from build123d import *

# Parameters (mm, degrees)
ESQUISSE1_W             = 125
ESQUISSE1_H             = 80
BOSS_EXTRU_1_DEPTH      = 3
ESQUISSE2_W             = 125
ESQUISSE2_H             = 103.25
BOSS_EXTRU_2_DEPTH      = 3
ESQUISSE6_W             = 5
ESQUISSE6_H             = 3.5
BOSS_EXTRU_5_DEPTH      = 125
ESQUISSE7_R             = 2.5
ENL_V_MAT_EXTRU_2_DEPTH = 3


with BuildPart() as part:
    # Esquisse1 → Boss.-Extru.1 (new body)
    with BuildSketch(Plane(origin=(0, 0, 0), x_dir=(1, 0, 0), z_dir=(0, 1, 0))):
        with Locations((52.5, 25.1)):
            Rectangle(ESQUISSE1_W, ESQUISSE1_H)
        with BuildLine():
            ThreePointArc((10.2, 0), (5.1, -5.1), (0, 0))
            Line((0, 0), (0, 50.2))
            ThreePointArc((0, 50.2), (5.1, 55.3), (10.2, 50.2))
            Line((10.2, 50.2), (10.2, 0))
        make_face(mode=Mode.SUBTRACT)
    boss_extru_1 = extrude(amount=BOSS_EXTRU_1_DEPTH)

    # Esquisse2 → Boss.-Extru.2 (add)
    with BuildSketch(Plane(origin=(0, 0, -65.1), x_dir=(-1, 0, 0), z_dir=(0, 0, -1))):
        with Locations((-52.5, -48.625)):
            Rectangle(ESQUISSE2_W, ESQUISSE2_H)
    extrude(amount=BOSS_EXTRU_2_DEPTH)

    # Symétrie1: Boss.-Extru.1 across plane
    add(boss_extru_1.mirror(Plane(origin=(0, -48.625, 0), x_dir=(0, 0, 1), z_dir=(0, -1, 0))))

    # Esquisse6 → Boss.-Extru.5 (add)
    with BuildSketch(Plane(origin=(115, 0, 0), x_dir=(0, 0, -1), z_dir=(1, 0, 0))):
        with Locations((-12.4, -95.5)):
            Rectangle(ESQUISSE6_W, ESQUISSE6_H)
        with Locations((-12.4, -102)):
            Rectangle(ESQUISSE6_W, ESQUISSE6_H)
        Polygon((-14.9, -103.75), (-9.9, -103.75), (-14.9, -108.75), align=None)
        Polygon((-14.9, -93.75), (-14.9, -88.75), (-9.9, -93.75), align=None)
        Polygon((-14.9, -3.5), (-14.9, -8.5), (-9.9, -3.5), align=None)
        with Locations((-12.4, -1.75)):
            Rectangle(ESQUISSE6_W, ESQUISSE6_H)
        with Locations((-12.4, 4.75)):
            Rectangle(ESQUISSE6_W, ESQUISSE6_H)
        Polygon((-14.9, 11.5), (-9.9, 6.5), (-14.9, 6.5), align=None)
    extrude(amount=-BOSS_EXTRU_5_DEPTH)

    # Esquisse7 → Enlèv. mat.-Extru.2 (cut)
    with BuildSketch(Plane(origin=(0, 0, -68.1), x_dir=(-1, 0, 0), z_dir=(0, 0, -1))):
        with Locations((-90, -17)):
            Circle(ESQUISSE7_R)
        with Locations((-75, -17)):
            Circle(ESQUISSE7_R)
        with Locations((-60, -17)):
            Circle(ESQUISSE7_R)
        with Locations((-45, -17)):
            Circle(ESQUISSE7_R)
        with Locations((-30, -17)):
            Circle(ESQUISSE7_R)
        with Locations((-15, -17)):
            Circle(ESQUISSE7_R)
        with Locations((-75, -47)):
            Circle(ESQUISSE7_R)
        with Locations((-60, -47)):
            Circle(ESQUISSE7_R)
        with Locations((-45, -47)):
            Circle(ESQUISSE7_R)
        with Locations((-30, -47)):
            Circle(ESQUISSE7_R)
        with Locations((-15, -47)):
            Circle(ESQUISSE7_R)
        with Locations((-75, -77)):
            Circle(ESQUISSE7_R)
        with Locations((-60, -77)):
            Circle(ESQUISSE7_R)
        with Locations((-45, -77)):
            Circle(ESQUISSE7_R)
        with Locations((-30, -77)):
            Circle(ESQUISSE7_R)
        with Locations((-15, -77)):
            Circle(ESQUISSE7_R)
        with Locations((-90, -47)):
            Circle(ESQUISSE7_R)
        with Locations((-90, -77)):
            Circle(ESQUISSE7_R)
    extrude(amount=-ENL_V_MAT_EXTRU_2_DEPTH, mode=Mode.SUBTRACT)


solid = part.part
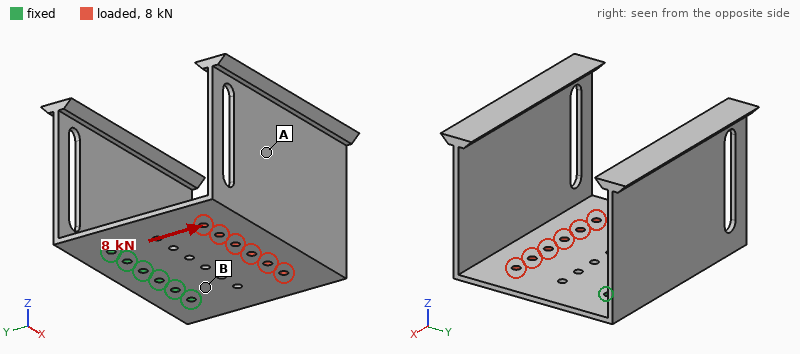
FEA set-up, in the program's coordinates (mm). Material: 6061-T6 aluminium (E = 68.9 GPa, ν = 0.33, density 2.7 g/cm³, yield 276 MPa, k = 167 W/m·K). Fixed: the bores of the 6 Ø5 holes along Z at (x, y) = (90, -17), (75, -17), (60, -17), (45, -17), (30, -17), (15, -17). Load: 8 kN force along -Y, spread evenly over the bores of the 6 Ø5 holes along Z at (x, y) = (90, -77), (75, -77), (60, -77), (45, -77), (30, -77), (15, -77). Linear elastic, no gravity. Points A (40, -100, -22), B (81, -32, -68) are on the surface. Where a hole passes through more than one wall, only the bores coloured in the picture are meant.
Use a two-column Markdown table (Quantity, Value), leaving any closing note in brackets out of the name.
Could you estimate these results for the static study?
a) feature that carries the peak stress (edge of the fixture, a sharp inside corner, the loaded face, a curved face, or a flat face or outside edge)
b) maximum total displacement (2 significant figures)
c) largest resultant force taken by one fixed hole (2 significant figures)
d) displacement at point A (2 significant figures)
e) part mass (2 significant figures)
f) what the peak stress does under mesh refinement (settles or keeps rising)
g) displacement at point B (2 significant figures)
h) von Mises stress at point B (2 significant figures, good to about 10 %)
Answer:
| Quantity | Value |
|---|---|
| feature that carries the peak stress | edge of the fixture |
| maximum total displacement | 31 µm |
| largest resultant force taken by one fixed hole | 1.9 kN |
| displacement at point A | 28 µm |
| part mass | 290 g |
| what the peak stress does under mesh refinement | keeps rising |
| displacement at point B | 6.5 µm |
| von Mises stress at point B | 27 MPa |
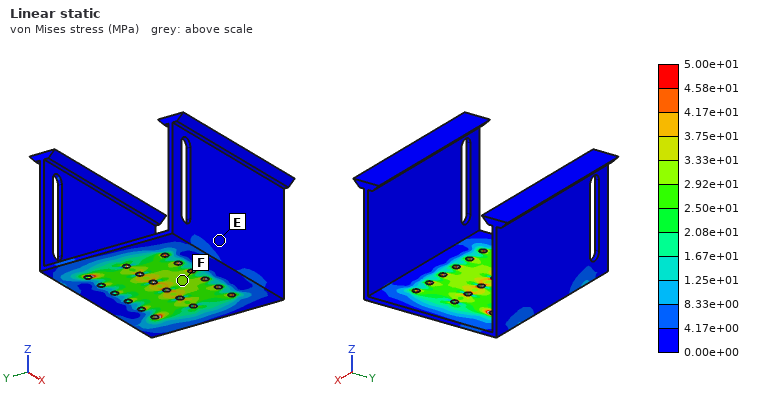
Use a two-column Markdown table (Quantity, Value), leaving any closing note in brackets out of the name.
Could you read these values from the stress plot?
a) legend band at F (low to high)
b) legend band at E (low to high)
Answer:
| Quantity | Value |
|---|---|
| legend band at F | 2.92e+01 to 3.33e+01 MPa |
| legend band at E | 0.00e+00 to 4.17e+00 MPa |
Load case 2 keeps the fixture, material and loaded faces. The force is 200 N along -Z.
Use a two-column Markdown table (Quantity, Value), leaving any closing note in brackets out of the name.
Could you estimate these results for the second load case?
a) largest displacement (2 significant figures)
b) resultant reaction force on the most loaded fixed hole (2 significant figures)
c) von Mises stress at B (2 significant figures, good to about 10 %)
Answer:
| Quantity | Value |
|---|---|
| largest displacement | 1.9 mm |
| resultant reaction force on the most loaded fixed hole | 70 N |
| von Mises stress at B | 44 MPa |
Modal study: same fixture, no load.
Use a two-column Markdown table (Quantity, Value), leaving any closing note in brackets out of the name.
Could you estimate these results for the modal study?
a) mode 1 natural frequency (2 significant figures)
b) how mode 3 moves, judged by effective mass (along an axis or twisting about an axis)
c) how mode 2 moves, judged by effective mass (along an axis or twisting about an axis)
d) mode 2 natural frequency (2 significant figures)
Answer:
| Quantity | Value |
|---|---|
| mode 1 natural frequency | 110 Hz |
| how mode 3 moves, judged by effective mass | along Y |
| how mode 2 moves, judged by effective mass | along X |
| mode 2 natural frequency | 190 Hz |
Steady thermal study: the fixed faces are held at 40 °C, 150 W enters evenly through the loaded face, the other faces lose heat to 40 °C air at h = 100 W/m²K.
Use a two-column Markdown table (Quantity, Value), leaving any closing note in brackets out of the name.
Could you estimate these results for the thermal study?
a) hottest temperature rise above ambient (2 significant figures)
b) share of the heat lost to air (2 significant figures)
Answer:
| Quantity | Value |
|---|---|
| hottest temperature rise above ambient | 68 K |
| share of the heat lost to air | 73 % |
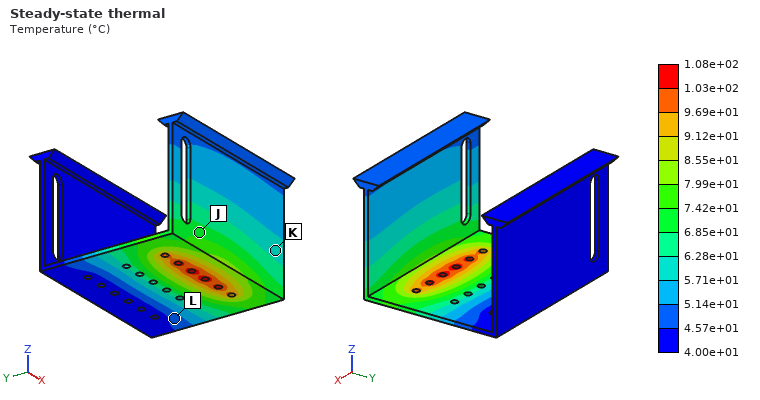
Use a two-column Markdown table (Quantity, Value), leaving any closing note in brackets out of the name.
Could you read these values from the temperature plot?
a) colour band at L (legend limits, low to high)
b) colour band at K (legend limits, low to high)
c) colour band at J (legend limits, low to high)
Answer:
| Quantity | Value |
|---|---|
| colour band at L | 4.57e+01 to 5.14e+01 °C |
| colour band at K | 5.71e+01 to 6.28e+01 °C |
| colour band at J | 6.85e+01 to 7.42e+01 °C |
